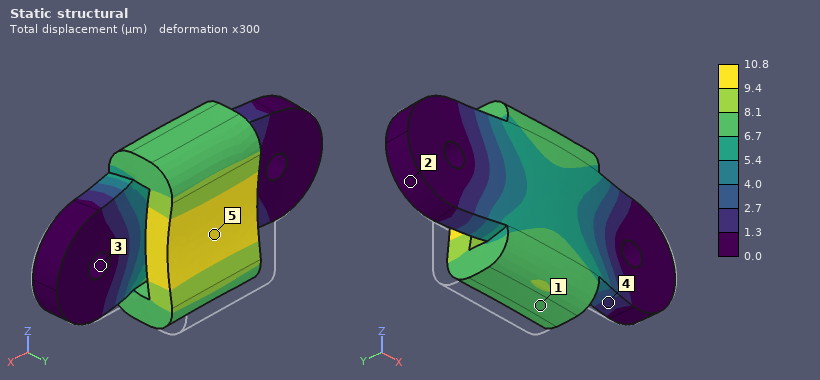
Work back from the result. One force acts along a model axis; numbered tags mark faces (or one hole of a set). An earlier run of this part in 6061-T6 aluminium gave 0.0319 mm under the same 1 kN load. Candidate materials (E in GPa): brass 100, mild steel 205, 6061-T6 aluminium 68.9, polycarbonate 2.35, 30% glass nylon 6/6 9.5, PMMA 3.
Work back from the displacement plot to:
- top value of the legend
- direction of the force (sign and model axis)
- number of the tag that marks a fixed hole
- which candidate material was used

10.8 µm
-Y
3
mild steel
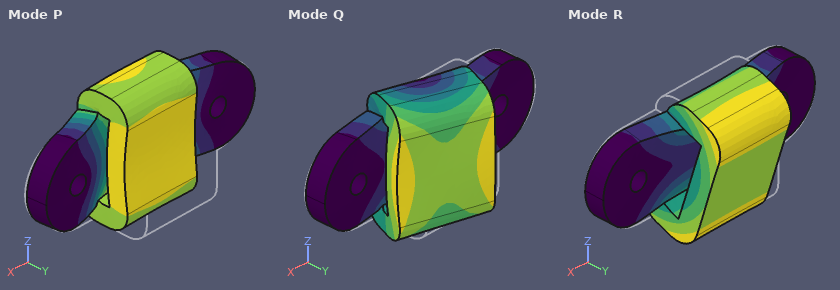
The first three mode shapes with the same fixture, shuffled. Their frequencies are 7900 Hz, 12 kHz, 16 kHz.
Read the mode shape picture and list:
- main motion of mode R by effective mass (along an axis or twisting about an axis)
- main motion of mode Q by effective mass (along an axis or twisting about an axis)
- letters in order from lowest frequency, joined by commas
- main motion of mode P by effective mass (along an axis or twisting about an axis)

along Z
along X
R, P, Q
along Y
